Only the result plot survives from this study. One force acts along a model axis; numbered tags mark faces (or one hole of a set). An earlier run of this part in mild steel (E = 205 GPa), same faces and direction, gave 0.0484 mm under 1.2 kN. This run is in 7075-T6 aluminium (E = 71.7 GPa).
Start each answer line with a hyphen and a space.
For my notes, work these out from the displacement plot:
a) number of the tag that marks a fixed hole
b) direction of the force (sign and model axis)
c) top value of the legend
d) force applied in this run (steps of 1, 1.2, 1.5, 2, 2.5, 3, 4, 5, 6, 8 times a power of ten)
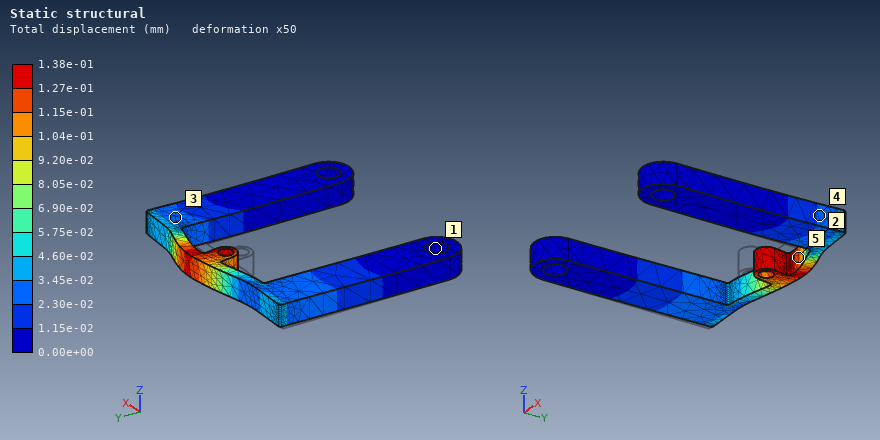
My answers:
- 1
- +Y
- 1.38e-01 mm
- 1.2 kN
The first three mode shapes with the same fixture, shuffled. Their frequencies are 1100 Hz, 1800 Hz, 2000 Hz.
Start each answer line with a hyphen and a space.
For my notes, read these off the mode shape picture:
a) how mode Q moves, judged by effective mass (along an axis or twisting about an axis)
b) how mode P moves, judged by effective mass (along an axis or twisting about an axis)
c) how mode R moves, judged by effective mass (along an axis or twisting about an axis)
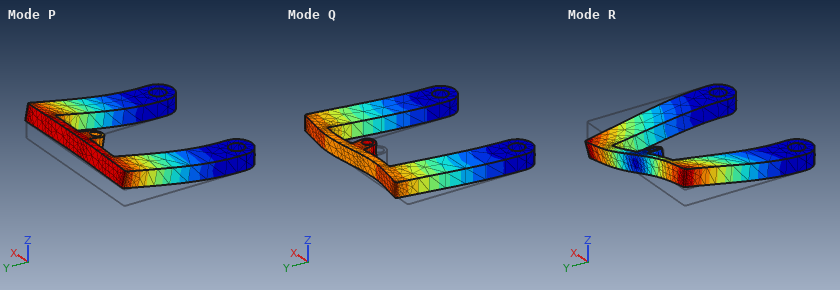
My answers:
- along X
- along Z
- twisting about Y
